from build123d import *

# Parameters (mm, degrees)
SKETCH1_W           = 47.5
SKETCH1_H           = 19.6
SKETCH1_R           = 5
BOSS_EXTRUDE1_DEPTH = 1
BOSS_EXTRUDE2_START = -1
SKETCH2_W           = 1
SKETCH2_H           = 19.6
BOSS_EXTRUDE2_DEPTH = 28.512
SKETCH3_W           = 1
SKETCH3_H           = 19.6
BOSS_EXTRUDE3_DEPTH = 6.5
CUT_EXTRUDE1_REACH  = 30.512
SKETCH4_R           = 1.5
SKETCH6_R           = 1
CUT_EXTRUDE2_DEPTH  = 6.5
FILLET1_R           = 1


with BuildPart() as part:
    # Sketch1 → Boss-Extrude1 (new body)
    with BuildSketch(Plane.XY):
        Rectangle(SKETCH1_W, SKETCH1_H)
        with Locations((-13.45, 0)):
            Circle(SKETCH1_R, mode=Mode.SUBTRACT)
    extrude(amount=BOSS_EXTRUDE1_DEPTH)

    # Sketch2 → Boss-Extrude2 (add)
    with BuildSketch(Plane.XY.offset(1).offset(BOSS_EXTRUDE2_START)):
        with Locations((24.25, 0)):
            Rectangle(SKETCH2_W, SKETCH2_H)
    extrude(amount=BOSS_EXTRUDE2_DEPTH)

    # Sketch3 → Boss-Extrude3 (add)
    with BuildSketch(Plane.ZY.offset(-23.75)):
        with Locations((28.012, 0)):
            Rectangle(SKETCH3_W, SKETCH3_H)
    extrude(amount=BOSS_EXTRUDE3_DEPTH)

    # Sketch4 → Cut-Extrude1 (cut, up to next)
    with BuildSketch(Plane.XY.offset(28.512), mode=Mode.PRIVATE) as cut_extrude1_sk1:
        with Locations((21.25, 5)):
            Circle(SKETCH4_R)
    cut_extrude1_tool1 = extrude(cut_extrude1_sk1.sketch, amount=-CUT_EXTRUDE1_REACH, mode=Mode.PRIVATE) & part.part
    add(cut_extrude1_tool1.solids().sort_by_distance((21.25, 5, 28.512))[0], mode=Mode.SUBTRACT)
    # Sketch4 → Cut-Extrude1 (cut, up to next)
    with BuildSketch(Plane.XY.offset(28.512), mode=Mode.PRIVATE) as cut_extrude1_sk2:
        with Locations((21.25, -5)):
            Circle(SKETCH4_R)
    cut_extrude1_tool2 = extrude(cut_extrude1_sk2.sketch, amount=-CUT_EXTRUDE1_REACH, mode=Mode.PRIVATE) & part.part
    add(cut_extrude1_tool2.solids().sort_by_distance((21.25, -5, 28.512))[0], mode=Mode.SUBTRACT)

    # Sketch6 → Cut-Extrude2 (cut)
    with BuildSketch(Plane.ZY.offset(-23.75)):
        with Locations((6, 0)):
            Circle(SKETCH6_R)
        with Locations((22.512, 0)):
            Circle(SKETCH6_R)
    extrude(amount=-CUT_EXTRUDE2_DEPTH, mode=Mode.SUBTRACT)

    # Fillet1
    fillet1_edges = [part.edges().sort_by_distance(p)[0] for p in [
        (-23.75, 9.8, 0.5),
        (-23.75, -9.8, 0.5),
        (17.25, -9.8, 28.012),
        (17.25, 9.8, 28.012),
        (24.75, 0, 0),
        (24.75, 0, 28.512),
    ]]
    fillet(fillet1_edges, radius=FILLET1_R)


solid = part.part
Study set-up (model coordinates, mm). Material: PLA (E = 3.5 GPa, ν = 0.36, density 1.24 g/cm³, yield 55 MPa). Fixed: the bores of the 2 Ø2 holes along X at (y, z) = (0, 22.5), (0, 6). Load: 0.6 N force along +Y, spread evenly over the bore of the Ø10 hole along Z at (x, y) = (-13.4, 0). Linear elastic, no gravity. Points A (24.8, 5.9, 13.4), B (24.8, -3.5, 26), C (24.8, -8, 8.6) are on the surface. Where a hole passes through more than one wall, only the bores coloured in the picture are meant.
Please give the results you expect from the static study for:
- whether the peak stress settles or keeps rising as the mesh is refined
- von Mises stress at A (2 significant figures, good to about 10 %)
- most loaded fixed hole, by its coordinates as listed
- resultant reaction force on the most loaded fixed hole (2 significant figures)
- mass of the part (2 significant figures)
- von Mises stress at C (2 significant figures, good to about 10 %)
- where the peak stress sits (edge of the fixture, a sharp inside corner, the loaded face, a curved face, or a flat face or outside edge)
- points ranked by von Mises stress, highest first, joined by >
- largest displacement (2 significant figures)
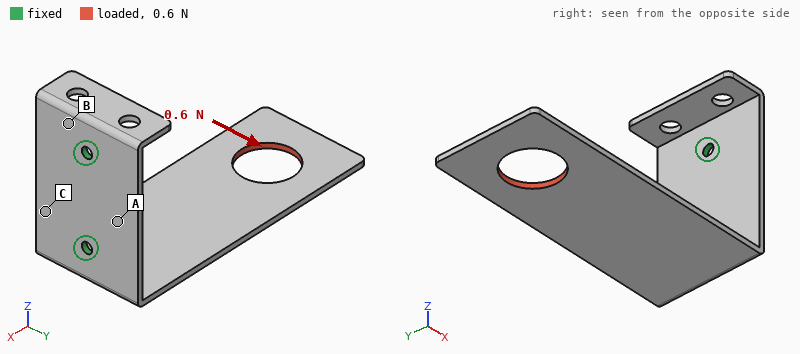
keeps rising
1.2 MPa
(0, 6)
0.76 N
1.9 g
2.3 MPa
edge of the fixture
C > A > B
0.63 mm
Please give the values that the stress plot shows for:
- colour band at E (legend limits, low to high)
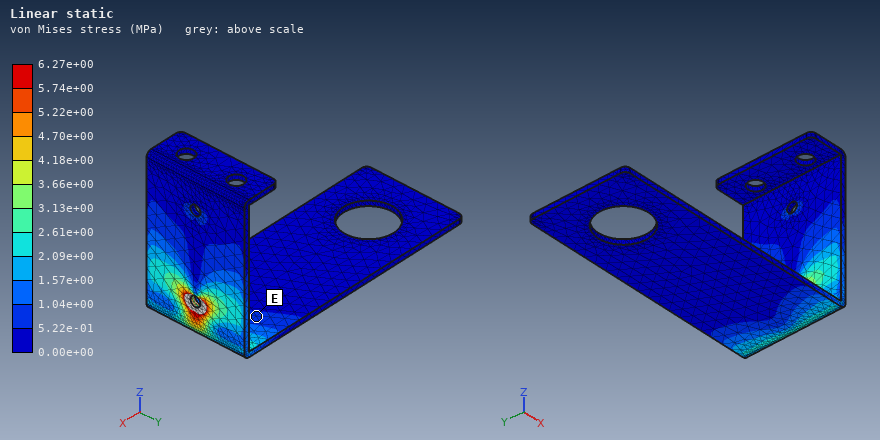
5.22e-01 to 1.04e+00 MPa
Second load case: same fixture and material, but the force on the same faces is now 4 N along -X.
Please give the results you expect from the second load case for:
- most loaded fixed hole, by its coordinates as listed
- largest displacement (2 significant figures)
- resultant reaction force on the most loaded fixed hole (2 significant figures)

(0, 6)
0.58 mm
4.3 N
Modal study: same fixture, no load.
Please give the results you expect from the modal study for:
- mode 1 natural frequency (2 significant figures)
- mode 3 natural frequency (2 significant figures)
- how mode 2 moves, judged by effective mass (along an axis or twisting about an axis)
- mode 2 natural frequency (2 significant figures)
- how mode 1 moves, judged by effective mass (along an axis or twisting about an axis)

110 Hz
570 Hz
along Y
240 Hz
along Z
